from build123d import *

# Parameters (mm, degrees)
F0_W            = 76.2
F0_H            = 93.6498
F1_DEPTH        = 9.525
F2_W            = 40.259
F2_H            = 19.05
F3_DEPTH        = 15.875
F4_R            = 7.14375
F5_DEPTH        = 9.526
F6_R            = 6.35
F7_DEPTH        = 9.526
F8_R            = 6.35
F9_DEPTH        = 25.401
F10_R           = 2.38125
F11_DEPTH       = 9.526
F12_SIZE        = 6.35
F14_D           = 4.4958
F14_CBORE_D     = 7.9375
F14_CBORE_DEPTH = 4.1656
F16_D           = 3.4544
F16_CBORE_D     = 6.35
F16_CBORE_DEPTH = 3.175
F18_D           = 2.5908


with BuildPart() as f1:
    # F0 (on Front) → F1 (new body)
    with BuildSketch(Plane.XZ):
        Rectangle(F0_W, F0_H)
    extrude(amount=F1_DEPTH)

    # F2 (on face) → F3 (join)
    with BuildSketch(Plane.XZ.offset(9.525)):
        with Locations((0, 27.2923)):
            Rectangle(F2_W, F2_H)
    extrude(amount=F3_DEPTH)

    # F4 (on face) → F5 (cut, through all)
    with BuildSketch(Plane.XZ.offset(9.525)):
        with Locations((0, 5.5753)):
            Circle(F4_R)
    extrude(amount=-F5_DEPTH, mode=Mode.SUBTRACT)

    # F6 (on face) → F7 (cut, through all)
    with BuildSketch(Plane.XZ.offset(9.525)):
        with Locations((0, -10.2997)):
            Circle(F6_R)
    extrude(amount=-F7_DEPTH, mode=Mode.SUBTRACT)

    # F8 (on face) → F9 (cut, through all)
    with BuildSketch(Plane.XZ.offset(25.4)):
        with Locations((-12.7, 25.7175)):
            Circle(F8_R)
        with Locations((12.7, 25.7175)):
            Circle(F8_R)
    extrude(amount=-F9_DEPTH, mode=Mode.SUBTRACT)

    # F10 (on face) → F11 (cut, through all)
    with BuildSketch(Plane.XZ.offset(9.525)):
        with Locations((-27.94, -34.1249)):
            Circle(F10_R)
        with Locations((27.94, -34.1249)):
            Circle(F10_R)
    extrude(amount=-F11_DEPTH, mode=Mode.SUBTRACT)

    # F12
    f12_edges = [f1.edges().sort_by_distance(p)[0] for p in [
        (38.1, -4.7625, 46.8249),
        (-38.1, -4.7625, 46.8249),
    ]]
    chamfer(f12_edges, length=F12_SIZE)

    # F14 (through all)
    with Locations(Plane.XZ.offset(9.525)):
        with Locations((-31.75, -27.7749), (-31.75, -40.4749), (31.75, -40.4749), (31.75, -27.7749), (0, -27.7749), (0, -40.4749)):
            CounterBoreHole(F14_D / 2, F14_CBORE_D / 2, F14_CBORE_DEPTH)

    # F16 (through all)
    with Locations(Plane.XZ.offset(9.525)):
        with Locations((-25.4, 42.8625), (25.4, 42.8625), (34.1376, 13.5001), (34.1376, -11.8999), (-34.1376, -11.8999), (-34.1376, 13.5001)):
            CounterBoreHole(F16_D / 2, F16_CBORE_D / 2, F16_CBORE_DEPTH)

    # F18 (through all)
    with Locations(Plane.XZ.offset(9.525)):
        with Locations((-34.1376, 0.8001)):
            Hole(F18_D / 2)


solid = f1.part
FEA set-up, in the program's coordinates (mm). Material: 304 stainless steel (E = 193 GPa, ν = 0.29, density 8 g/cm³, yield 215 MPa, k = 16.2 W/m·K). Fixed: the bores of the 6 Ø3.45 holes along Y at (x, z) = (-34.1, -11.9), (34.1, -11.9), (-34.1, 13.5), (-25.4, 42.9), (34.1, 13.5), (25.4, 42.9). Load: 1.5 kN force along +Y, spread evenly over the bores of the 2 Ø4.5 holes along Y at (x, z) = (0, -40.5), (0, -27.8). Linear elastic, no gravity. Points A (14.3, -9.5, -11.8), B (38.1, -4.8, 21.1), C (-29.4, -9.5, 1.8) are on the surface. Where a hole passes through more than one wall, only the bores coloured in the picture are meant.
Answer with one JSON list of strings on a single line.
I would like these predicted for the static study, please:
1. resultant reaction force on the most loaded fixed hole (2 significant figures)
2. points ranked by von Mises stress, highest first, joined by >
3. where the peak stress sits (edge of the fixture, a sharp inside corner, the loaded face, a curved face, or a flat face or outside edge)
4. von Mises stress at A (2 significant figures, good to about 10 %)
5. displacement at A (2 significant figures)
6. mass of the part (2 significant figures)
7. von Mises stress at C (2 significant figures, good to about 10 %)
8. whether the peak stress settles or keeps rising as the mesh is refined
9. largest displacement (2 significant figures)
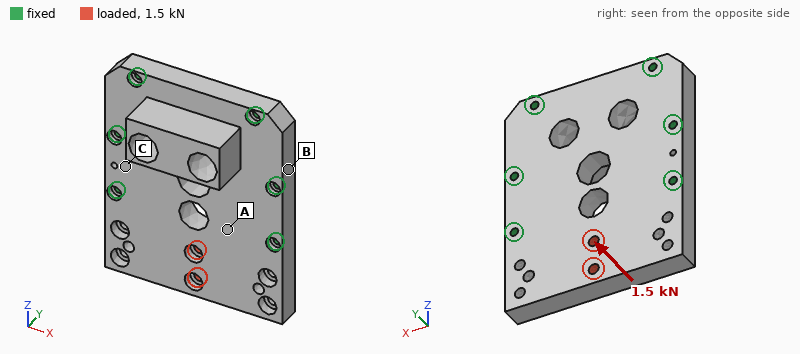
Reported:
["1.3 kN", "A > C > B", "edge of the fixture", "28 MPa", "8.5 µm", "540 g", "19 MPa", "keeps rising", "43 µm"]
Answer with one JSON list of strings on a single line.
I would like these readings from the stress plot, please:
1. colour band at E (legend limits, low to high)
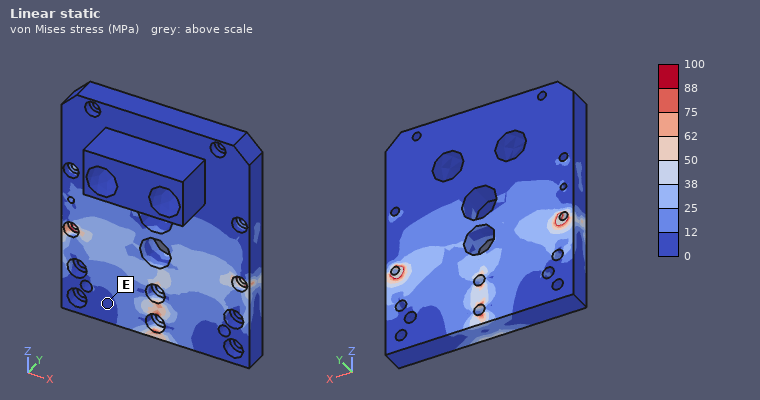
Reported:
["0 to 12 MPa"]
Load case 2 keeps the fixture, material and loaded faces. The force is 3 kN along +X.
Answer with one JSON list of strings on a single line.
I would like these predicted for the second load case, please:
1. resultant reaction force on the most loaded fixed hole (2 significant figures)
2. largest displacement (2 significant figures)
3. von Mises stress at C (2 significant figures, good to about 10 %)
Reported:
["1.5 kN", "4.2 µm", "4.4 MPa"]
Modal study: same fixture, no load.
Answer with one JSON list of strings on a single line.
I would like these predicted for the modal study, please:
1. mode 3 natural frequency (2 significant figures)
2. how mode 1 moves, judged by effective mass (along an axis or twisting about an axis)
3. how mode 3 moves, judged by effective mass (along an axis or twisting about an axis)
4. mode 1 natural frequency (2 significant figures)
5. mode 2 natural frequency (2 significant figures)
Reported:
["7900 Hz", "along Y", "along Y", "3500 Hz", "7000 Hz"]
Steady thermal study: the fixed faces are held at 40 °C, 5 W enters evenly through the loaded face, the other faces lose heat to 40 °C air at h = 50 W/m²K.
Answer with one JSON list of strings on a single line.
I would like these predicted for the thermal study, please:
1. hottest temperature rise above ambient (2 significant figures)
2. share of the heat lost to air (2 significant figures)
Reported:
["19 K", "62 %"]
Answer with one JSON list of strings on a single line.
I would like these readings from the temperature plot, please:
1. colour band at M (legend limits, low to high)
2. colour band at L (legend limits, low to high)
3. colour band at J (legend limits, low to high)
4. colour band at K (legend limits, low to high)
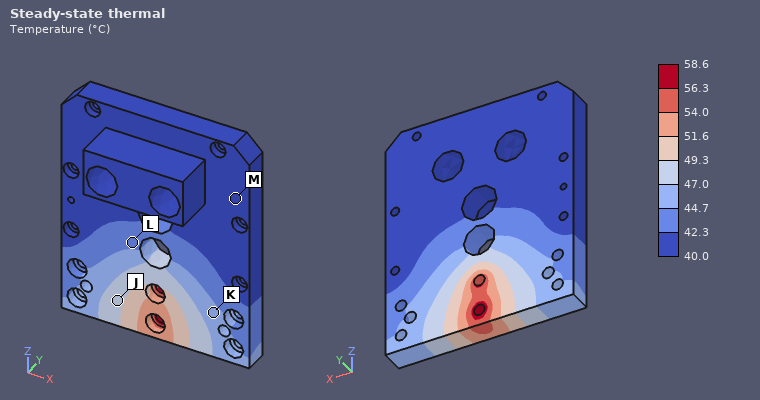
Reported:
["40.0 to 42.3 °C", "42.3 to 44.7 °C", "47.0 to 49.3 °C", "44.7 to 47.0 °C"]
